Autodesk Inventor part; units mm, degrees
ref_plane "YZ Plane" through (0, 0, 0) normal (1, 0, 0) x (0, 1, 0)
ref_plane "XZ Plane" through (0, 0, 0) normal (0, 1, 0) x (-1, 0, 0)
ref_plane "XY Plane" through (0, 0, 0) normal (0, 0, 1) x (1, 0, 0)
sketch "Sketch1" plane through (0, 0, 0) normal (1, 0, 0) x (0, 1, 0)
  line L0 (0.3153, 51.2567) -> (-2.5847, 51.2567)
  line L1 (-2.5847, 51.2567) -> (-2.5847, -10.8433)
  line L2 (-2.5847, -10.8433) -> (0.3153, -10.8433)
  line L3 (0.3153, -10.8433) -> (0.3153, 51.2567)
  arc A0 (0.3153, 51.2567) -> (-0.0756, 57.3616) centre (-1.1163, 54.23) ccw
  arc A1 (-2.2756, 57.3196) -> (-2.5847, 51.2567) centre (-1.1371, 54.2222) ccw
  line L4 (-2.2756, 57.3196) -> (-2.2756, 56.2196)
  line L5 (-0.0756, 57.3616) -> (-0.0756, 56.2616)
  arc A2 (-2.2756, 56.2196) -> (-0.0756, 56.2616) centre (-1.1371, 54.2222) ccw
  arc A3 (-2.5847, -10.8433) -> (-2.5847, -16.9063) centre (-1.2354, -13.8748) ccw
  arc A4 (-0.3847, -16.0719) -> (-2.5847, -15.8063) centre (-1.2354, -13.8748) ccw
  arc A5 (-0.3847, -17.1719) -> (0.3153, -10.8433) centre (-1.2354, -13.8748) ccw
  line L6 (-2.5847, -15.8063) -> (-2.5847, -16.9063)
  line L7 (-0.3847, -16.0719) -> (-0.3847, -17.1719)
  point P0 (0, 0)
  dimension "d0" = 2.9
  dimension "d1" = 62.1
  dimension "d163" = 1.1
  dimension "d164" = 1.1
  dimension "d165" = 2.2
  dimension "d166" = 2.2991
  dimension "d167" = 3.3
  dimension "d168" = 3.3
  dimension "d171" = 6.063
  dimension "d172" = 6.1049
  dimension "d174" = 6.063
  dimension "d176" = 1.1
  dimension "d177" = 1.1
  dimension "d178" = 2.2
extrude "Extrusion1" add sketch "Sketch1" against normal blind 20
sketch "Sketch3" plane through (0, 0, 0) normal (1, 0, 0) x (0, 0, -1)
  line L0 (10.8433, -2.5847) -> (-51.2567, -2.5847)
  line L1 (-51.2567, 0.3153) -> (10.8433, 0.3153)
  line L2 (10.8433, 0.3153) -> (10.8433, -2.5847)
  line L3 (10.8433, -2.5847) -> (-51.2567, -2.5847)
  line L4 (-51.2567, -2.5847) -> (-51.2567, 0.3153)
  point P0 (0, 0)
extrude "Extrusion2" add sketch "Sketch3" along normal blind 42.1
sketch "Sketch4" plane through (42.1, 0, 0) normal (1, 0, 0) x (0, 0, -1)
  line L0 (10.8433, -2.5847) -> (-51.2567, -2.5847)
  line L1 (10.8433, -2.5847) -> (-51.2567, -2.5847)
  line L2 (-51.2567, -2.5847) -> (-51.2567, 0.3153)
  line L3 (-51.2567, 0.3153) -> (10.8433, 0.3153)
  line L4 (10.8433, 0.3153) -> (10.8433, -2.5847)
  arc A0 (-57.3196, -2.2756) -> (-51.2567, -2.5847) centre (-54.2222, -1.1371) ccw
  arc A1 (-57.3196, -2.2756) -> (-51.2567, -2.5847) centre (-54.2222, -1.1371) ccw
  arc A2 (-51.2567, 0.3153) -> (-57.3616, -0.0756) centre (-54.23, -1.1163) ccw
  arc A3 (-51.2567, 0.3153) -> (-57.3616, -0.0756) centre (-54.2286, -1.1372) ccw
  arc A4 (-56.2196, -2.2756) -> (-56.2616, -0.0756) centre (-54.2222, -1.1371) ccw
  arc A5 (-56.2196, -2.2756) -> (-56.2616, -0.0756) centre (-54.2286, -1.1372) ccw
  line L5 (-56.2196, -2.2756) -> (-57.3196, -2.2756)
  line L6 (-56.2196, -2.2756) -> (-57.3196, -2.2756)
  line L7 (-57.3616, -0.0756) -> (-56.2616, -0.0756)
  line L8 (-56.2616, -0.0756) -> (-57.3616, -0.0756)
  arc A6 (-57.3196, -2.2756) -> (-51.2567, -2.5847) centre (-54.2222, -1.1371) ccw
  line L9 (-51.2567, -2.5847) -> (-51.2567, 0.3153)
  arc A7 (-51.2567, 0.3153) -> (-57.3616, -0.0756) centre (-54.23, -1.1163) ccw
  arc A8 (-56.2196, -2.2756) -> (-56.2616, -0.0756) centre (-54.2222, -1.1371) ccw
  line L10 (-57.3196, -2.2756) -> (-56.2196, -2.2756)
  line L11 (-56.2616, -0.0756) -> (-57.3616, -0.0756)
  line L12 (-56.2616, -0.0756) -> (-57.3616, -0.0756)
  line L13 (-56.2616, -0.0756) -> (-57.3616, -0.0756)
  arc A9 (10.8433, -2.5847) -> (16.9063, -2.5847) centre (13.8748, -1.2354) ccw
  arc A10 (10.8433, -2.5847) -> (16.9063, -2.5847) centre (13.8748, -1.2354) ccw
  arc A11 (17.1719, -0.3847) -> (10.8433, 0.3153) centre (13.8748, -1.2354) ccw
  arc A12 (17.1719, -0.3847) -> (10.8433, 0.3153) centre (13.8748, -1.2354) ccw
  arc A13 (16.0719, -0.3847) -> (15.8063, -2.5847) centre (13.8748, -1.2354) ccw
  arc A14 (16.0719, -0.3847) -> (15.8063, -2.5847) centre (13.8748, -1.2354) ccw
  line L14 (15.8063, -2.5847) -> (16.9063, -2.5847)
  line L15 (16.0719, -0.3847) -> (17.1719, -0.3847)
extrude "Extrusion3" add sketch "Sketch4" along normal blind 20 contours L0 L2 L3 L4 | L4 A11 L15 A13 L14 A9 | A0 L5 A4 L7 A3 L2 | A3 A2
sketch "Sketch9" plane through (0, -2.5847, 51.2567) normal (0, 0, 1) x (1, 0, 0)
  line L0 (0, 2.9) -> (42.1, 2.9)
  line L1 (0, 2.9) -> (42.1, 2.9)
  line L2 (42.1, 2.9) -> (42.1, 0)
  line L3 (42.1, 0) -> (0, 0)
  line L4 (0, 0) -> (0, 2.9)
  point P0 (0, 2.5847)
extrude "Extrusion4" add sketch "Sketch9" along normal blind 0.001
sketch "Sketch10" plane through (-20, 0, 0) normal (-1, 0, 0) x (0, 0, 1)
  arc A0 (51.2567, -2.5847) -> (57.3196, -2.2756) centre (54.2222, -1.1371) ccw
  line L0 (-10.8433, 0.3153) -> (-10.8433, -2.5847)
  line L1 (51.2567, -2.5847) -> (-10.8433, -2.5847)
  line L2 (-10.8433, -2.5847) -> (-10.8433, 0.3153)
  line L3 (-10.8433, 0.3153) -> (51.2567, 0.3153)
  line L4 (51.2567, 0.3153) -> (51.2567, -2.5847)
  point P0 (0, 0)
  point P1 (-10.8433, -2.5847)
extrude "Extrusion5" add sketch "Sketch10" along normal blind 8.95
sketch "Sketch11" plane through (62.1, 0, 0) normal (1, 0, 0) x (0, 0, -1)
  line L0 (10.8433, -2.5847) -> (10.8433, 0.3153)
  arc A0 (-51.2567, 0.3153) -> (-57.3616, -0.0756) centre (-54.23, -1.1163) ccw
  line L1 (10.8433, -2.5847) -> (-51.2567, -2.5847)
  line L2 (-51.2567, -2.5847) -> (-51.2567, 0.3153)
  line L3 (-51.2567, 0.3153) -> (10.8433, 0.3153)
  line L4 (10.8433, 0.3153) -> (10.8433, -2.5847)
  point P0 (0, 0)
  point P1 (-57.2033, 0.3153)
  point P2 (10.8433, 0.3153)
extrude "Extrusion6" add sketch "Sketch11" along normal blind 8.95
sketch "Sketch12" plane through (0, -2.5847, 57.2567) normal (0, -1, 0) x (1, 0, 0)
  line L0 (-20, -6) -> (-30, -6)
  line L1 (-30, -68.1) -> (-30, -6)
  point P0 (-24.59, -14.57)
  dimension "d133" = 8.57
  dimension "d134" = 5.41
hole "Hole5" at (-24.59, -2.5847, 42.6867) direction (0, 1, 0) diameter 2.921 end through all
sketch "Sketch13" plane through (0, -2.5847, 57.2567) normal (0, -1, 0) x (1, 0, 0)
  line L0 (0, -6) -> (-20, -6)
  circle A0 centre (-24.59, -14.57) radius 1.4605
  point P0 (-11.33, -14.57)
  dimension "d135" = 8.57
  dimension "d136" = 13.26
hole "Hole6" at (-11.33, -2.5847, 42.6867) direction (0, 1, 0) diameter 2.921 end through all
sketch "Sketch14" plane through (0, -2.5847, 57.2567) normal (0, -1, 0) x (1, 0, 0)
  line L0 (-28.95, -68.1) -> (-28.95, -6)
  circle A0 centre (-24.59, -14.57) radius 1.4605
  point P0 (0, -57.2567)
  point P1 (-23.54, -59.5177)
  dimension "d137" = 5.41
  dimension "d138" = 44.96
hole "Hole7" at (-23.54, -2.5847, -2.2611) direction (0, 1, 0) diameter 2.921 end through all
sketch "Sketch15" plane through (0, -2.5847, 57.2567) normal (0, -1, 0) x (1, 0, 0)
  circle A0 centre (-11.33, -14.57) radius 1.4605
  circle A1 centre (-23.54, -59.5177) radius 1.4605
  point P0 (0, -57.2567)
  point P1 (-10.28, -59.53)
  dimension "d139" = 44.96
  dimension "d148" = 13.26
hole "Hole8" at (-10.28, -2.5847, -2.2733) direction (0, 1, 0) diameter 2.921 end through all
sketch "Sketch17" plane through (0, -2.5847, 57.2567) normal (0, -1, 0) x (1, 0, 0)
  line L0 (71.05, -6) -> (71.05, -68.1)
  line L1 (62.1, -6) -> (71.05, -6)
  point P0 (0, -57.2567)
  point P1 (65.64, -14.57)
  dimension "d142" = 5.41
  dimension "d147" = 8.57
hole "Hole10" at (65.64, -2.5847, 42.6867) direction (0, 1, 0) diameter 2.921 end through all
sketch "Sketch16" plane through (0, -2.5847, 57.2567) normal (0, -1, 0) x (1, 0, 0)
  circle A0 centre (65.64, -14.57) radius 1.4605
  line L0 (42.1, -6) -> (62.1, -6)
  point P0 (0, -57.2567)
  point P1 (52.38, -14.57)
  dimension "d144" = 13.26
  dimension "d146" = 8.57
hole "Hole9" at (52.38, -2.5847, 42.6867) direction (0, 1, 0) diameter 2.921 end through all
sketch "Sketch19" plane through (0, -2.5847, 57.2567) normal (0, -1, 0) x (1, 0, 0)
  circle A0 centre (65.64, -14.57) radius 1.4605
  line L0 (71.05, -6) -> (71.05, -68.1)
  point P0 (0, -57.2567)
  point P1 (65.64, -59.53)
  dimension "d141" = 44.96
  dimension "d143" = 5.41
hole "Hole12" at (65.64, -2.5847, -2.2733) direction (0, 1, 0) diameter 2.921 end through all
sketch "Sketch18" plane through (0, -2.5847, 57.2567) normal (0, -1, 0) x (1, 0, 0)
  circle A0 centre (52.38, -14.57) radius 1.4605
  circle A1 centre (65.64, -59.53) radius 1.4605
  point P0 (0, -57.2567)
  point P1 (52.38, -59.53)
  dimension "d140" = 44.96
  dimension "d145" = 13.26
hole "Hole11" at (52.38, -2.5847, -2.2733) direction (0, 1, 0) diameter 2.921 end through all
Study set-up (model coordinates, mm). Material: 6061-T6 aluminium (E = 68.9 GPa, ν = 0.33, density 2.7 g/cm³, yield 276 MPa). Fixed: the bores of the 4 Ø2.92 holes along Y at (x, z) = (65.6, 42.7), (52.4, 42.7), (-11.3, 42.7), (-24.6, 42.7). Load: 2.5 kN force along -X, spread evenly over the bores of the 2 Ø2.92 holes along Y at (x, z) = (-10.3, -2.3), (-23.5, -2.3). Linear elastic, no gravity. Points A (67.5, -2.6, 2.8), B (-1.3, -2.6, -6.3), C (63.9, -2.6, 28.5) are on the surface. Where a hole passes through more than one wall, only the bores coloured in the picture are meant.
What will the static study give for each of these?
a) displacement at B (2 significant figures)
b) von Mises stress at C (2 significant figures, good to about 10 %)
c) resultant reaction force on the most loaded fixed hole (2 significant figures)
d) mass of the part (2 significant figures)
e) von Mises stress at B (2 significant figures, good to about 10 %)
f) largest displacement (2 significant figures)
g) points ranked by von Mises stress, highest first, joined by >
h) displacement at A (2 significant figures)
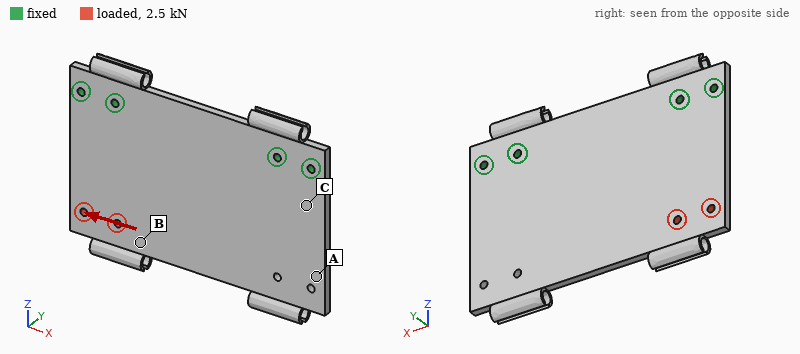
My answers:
31 µm
15 MPa
1.2 kN
51 g
34 MPa
43 µm
B > C > A
17 µm
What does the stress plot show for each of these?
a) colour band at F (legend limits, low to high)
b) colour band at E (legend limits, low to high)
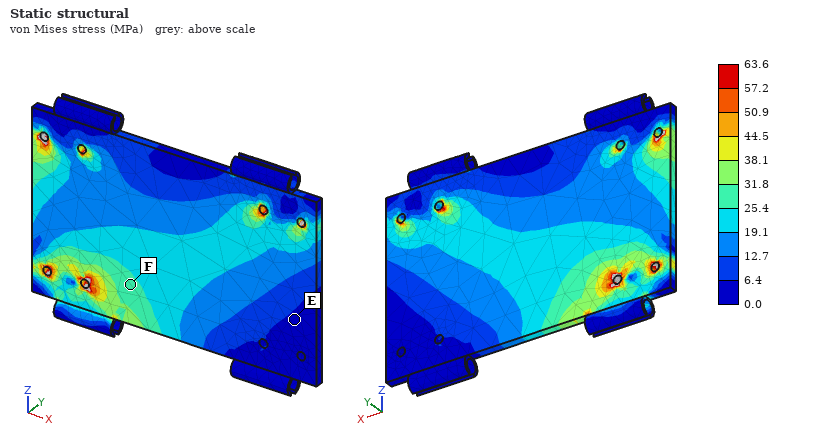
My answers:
25.4 to 31.8 MPa
0.0 to 6.4 MPa
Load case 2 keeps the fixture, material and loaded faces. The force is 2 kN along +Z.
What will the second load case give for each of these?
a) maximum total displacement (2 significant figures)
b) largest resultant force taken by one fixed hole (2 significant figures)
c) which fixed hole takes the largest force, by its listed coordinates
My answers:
22 µm
1.1 kN
(-11.3, 42.7)
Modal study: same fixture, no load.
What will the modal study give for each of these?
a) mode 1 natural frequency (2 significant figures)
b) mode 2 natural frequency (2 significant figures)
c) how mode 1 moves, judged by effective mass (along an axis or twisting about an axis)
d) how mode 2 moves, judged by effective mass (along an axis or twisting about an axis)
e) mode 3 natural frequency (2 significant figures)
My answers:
660 Hz
1200 Hz
along Y
twisting about Z
2400 Hz
